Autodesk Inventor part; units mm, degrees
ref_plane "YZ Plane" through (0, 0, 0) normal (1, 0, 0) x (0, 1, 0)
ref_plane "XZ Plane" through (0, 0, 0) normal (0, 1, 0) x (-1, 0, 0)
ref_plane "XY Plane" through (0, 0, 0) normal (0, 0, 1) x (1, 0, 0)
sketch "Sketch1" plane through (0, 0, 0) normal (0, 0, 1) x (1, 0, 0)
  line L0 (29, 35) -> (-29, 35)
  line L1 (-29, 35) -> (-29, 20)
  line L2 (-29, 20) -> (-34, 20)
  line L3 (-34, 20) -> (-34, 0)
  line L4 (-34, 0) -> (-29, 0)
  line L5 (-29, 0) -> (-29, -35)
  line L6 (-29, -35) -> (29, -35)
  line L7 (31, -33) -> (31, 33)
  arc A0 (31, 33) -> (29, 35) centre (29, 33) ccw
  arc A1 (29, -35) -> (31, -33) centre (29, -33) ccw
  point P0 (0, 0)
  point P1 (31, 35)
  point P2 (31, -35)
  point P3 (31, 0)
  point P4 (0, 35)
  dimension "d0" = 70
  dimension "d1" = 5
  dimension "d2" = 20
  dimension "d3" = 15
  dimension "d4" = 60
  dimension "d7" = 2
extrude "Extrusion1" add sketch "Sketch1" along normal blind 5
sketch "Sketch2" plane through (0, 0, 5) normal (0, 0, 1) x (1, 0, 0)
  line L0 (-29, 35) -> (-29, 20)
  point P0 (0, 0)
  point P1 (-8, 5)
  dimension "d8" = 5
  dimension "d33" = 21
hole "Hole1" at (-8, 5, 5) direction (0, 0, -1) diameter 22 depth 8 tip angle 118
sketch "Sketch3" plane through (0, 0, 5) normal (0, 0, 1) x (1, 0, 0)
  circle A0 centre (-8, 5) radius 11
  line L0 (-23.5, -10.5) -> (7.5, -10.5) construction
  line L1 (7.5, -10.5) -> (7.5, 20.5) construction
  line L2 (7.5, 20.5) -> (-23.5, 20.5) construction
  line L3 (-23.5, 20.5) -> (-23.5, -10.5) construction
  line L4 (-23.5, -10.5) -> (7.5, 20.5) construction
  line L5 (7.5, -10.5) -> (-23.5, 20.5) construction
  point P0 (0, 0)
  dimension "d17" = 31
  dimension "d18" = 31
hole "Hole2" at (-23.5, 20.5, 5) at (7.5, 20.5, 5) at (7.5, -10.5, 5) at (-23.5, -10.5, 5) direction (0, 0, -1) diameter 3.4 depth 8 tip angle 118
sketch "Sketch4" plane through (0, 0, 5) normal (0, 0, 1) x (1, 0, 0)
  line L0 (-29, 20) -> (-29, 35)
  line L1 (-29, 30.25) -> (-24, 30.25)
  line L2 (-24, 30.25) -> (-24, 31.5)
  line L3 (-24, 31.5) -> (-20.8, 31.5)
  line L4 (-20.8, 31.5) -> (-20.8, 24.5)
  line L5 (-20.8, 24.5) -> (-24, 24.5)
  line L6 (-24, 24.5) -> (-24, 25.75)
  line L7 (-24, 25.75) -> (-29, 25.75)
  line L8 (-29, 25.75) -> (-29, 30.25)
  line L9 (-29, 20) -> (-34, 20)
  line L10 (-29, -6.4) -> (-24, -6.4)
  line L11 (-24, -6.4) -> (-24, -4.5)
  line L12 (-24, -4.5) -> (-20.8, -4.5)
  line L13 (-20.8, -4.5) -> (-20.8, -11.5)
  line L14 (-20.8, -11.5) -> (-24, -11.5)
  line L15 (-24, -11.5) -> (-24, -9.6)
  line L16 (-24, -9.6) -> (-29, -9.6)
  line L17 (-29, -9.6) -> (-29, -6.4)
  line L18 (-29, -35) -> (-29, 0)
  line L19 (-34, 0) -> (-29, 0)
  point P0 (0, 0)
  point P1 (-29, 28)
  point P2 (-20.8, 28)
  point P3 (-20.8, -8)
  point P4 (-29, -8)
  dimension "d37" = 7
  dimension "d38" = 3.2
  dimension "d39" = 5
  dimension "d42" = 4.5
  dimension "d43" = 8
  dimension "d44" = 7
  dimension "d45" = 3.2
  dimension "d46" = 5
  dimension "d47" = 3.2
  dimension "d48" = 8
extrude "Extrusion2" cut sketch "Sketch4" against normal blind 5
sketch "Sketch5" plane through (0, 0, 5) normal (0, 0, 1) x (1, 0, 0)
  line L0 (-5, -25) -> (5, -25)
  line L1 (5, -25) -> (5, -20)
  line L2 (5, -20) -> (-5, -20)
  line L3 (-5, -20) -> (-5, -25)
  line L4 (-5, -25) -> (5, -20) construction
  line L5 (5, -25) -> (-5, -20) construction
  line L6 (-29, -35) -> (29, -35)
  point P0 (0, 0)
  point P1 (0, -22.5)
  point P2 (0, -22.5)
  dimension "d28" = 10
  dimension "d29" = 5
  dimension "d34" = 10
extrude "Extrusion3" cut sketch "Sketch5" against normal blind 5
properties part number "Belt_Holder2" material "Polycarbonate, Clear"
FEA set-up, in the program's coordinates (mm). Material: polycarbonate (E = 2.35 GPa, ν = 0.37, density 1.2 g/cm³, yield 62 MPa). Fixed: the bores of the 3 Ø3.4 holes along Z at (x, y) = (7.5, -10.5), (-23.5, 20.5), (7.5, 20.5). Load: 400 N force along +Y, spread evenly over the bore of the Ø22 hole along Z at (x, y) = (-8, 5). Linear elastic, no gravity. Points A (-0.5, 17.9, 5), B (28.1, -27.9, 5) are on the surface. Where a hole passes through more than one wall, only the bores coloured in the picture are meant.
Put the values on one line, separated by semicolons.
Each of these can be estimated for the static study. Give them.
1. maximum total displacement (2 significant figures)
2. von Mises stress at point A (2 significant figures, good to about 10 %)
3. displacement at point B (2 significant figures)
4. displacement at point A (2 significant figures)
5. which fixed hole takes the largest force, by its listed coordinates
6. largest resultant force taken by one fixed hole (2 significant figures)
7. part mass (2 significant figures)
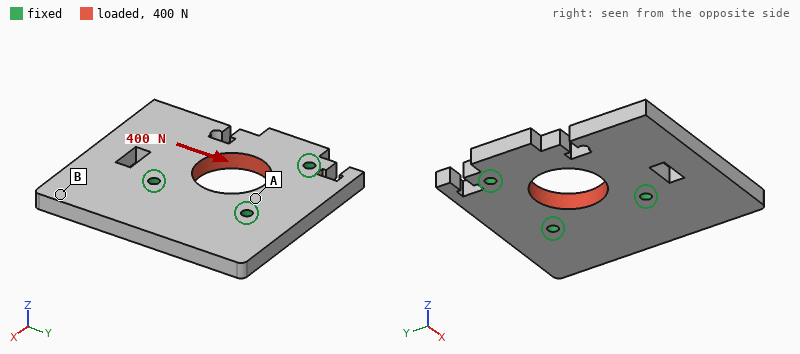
48 µm; 1.2 MPa; 12 µm; 9.5 µm; (-23.5, 20.5); 180 N; 23 g
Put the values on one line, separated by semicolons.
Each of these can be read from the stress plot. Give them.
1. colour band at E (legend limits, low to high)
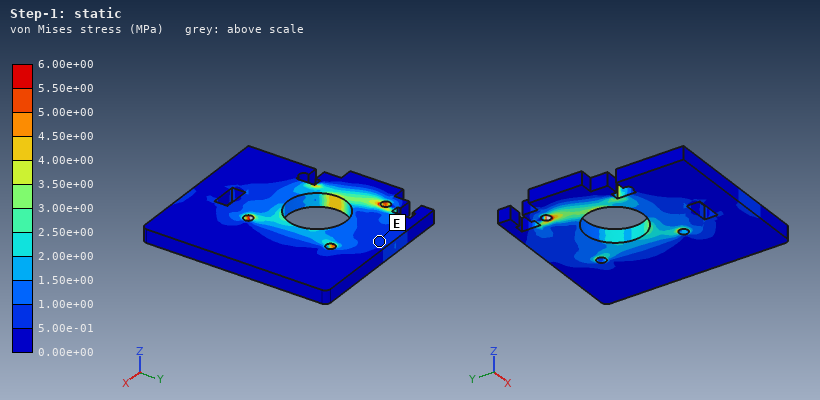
5.00e-01 to 1.00e+00 MPa
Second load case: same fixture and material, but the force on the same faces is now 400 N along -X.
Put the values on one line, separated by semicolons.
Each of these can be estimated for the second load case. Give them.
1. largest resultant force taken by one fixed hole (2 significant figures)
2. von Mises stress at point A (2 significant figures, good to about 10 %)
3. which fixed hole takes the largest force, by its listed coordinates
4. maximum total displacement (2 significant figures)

190 N; 1.8 MPa; (7.5, -10.5); 46 µm
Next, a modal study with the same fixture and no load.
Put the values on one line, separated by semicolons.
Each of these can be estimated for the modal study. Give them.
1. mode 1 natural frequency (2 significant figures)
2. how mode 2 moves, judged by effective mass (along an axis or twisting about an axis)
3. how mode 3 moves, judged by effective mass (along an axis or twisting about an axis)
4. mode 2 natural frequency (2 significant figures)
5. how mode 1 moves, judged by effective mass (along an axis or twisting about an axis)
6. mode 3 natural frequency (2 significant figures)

780 Hz; along Z; along Z; 1400 Hz; along Z; 1800 Hz
